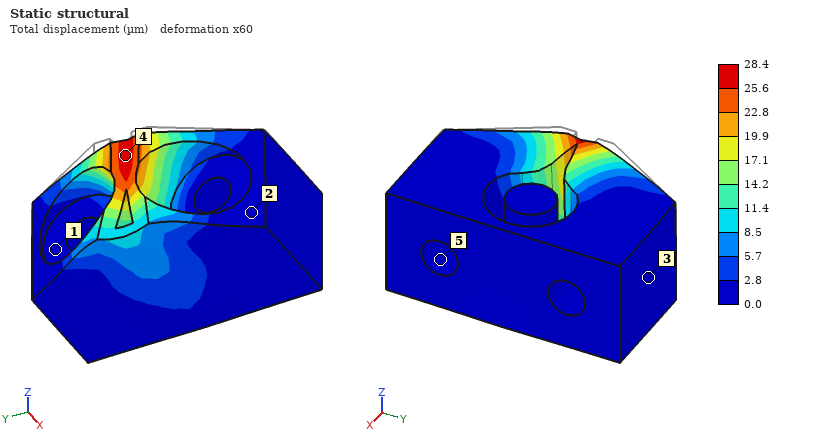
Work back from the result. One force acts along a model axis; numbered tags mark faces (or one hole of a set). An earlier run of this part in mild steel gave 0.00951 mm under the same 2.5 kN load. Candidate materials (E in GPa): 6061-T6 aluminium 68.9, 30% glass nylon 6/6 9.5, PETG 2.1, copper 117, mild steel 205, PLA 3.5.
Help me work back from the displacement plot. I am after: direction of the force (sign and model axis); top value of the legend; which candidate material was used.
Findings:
+X
28.4 µm
6061-T6 aluminium
